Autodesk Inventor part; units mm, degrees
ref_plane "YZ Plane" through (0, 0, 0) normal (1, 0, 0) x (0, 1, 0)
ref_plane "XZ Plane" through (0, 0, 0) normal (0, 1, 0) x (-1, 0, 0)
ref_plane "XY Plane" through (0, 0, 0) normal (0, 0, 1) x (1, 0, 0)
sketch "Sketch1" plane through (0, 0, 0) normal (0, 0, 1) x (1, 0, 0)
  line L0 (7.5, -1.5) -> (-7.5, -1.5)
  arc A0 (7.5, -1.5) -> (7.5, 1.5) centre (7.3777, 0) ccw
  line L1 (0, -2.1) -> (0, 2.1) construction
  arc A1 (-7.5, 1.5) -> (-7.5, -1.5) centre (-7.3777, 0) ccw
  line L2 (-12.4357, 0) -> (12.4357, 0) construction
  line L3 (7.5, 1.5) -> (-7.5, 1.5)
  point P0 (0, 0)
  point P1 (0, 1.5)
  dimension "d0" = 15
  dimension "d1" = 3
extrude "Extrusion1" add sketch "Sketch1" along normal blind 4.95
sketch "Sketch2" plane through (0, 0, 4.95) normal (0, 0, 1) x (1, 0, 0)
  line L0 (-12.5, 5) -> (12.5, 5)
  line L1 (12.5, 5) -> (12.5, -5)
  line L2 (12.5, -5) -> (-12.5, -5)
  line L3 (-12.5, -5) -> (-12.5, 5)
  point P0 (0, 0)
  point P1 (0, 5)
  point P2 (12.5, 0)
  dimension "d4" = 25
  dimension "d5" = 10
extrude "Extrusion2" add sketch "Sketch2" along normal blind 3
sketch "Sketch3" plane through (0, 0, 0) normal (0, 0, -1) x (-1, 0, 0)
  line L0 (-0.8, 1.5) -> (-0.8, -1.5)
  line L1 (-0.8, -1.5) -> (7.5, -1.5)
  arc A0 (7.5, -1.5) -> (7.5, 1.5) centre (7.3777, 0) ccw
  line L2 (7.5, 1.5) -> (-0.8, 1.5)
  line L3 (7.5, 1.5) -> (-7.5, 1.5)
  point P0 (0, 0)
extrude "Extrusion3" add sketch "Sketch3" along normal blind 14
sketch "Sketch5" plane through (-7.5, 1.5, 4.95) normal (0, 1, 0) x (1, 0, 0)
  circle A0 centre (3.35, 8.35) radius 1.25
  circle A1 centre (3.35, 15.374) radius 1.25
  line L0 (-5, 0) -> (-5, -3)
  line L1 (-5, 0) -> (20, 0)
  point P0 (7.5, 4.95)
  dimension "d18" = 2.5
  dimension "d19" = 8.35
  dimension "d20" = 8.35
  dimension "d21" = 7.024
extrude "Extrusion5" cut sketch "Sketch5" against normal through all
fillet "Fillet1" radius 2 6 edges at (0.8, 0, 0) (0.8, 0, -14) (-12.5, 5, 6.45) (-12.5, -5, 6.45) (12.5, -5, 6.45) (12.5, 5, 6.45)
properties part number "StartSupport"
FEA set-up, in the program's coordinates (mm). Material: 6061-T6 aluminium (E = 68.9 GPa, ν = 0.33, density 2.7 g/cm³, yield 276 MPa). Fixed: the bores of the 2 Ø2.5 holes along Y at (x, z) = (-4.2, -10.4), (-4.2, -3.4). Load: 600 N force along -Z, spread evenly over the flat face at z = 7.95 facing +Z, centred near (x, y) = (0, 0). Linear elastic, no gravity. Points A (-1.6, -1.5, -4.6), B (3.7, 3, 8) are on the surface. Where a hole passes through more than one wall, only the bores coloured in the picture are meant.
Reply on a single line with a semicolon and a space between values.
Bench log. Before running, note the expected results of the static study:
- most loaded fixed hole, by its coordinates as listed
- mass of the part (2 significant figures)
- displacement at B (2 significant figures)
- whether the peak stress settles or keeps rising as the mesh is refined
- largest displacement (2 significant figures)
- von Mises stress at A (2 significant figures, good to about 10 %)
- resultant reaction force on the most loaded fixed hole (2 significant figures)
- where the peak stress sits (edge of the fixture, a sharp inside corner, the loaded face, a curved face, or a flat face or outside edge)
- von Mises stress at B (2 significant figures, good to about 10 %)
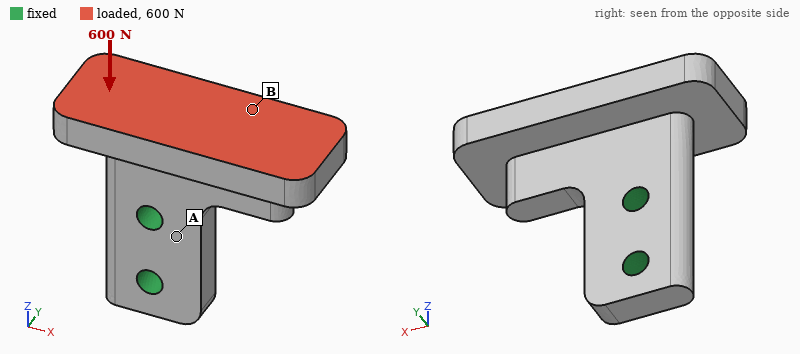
(-4.2, -3.4); 3.7 g; 23 µm; keeps rising; 41 µm; 38 MPa; 510 N; edge of the fixture; 16 MPa
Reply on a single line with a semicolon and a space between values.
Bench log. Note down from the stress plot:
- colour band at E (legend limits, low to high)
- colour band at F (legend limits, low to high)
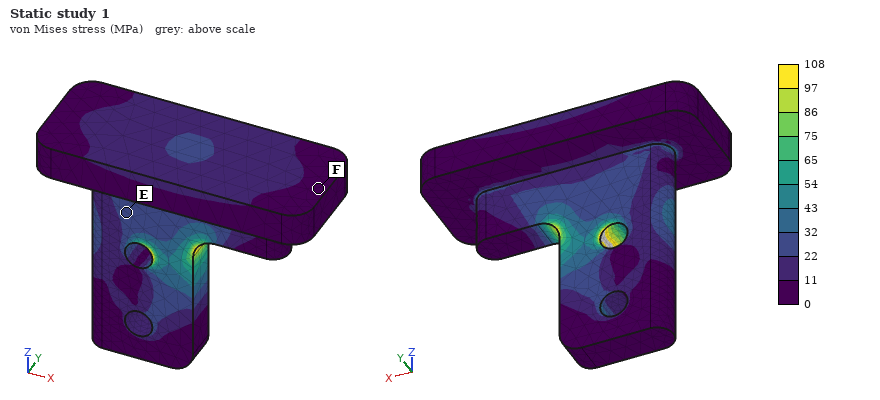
22 to 32 MPa; 0 to 11 MPa
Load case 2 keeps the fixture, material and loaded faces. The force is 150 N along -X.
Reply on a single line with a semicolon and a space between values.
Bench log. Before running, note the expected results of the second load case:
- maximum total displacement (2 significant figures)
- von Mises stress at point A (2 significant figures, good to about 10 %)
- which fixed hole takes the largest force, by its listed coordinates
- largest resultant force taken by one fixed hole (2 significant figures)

21 µm; 17 MPa; (-4.2, -3.4); 280 N
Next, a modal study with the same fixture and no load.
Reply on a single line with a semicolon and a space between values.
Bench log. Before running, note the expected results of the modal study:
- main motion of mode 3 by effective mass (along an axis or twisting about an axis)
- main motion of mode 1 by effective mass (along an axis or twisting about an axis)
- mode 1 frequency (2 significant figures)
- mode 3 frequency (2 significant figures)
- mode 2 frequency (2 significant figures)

along X; along Y; 5600 Hz; 11 kHz; 9000 Hz
